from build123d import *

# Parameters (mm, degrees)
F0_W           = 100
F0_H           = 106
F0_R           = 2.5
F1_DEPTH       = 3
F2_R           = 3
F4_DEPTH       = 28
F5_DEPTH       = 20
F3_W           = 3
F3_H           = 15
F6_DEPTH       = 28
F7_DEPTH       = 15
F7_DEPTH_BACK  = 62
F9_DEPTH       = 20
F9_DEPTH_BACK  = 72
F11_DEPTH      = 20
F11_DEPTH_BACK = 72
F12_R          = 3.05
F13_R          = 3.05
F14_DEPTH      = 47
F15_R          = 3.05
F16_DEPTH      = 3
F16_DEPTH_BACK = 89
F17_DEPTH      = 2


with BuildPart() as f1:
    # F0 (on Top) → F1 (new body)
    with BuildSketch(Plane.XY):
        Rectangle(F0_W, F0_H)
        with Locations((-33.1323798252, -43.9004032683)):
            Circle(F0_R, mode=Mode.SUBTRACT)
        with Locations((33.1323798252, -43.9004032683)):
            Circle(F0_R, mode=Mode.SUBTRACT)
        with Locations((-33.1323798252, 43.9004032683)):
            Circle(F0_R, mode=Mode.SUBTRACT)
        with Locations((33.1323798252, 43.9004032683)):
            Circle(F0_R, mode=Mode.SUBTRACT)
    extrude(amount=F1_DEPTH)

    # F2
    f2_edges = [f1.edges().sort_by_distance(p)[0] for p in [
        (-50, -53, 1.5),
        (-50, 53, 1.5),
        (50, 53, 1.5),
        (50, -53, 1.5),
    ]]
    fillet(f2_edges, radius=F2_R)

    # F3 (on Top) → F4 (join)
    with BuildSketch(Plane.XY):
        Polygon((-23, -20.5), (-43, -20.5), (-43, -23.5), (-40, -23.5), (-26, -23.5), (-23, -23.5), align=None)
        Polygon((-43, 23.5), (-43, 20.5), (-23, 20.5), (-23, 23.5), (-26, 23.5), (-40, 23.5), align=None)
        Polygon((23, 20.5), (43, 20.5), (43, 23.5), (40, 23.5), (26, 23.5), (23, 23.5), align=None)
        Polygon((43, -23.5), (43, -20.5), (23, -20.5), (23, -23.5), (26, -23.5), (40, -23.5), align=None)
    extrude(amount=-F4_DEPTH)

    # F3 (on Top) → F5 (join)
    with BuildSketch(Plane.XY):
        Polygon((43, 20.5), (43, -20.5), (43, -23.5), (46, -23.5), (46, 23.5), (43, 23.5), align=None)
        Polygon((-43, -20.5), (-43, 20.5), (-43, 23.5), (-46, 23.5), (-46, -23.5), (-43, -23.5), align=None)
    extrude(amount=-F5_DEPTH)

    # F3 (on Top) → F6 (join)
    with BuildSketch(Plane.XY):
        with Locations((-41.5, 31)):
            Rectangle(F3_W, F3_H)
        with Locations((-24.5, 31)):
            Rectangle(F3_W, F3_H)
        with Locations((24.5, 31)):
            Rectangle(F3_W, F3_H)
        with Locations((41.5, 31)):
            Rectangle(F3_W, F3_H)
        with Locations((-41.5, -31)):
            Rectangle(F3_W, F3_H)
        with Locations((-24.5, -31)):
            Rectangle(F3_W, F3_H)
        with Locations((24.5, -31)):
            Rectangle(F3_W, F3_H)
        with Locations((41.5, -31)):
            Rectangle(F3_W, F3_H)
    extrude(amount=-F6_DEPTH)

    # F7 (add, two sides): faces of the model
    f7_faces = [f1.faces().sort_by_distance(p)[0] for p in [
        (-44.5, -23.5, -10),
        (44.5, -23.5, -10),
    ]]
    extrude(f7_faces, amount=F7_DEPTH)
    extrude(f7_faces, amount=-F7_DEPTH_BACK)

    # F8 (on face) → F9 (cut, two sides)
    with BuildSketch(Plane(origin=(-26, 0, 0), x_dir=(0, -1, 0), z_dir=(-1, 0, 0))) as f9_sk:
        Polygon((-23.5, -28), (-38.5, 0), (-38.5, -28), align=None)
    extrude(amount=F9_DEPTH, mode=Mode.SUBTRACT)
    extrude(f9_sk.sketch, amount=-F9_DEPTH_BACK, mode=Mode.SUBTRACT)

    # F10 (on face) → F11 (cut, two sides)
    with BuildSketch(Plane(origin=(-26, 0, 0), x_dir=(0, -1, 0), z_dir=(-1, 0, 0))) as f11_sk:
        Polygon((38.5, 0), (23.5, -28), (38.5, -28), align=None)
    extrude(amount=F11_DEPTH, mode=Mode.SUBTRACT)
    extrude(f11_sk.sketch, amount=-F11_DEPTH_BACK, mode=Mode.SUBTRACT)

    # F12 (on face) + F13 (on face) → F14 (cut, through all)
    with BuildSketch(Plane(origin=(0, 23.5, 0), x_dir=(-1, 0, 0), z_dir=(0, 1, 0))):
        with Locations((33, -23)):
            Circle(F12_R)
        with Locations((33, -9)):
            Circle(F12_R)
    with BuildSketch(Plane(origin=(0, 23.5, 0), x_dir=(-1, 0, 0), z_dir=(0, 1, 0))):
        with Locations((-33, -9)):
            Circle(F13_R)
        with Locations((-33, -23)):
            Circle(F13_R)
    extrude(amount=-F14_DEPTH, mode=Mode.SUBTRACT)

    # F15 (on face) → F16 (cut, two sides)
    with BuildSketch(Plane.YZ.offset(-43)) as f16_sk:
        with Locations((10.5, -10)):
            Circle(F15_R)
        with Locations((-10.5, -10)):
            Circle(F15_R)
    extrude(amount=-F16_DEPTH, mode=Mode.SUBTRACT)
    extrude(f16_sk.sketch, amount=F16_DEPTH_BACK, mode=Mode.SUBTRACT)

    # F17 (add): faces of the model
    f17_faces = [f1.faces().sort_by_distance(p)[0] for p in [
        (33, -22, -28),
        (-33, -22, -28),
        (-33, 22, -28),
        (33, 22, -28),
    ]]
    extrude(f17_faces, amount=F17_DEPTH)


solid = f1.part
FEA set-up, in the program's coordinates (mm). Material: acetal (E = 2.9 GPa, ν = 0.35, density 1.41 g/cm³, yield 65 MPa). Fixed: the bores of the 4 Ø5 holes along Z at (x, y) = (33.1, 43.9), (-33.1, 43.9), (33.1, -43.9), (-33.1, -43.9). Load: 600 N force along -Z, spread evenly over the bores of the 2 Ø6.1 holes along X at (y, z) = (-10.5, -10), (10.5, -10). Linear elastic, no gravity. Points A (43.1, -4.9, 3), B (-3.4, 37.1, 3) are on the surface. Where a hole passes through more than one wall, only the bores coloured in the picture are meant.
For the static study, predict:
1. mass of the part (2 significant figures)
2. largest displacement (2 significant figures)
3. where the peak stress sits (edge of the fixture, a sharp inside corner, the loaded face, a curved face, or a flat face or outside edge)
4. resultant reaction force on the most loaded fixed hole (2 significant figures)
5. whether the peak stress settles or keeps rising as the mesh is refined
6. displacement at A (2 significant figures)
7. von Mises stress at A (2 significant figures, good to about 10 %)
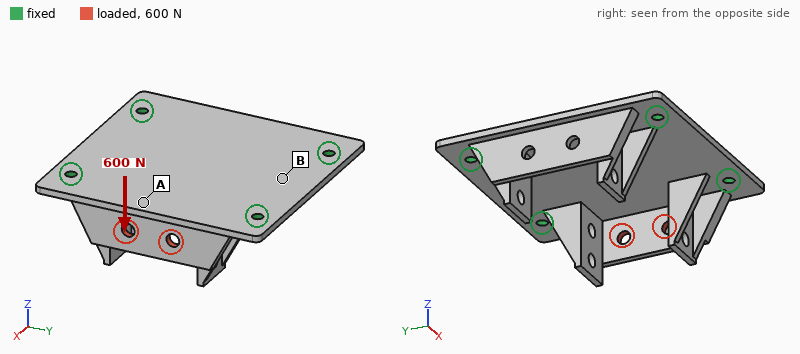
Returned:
71 g
1.8 mm
edge of the fixture
440 N
keeps rising
1.1 mm
8.4 MPa
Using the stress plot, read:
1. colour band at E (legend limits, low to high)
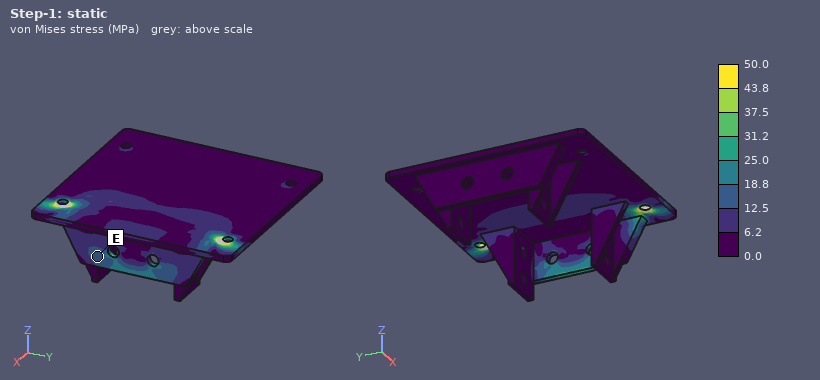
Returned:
12.5 to 18.8 MPa
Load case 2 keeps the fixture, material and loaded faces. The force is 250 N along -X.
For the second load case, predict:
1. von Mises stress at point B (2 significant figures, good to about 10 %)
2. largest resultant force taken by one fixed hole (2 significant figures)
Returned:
2.0 MPa
69 N
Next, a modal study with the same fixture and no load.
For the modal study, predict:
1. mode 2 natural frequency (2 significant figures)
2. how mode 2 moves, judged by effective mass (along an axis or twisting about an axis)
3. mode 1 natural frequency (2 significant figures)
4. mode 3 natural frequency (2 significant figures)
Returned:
880 Hz
along X
570 Hz
920 Hz
